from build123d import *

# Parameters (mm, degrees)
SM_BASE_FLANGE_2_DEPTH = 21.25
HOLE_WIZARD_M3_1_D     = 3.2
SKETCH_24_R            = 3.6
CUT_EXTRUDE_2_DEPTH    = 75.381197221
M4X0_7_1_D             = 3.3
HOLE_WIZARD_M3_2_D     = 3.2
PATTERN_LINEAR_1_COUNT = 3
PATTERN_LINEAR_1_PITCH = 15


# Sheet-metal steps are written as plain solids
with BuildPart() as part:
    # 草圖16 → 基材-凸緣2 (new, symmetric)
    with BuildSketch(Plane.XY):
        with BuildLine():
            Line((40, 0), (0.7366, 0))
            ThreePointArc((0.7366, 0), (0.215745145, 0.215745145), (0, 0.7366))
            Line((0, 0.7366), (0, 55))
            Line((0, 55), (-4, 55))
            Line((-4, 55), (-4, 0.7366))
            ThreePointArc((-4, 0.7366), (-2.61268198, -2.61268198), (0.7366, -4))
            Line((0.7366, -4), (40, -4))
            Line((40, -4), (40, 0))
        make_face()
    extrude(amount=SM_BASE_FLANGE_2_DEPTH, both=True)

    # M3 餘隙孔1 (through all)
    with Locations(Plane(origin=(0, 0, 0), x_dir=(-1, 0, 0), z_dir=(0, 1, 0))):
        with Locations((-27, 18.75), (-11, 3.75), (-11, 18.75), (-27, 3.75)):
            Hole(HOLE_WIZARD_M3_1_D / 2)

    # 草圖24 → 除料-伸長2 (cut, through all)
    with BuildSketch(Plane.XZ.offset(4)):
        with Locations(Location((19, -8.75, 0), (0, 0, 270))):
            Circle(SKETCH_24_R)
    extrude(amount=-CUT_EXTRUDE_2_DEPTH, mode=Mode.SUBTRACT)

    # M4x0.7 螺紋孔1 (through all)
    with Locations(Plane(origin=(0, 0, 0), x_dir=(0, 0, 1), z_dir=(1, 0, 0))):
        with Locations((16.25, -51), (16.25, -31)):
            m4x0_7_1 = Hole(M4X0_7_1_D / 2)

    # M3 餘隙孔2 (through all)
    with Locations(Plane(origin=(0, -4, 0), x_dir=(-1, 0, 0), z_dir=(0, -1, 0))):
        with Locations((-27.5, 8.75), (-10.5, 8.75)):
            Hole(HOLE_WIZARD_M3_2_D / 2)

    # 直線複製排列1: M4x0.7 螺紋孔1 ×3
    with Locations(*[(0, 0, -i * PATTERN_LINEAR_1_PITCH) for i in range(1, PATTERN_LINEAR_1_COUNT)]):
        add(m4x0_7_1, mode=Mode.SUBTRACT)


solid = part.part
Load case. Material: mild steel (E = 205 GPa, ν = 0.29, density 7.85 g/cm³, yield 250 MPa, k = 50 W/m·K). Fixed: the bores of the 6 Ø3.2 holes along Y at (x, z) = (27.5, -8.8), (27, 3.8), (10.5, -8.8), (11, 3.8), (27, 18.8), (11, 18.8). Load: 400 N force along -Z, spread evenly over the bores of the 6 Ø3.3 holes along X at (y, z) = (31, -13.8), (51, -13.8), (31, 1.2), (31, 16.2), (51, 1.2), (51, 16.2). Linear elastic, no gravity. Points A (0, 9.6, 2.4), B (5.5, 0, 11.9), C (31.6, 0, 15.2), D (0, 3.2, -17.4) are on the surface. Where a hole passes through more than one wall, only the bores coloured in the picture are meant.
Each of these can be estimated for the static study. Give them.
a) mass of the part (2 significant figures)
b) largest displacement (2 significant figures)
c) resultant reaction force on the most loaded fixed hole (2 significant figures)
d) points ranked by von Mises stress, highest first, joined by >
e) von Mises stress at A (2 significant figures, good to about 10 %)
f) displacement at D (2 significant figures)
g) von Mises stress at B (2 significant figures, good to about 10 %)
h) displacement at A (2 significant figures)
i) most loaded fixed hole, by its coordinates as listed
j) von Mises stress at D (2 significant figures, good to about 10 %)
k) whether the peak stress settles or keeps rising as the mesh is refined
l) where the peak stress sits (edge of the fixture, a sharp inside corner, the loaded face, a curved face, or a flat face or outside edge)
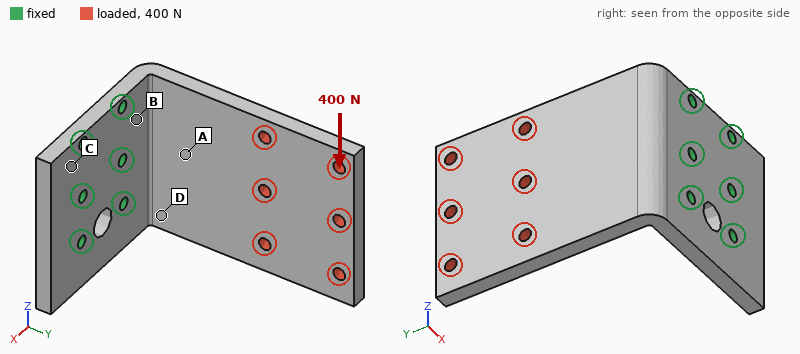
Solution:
130 g
65 µm
720 N
B > D > A > C
20 MPa
18 µm
53 MPa
12 µm
(10.5, -8.8)
39 MPa
keeps rising
edge of the fixture
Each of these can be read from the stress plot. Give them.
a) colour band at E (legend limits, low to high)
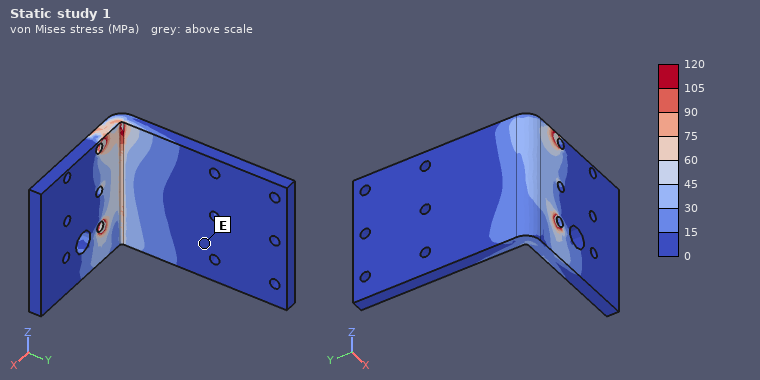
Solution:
0 to 15 MPa
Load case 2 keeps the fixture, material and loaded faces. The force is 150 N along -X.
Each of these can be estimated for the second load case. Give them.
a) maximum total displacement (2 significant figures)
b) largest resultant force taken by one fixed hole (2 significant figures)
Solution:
0.22 mm
89 N
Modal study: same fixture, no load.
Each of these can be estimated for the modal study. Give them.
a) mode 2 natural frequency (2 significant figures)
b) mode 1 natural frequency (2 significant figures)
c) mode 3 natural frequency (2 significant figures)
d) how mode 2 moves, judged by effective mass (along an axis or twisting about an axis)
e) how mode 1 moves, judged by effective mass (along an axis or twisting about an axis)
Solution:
2100 Hz
780 Hz
3100 Hz
along Z
along X
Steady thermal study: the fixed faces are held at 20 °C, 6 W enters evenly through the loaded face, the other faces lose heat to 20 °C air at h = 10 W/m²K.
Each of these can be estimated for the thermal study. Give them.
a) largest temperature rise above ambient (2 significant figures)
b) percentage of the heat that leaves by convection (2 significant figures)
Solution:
34 K
21 %
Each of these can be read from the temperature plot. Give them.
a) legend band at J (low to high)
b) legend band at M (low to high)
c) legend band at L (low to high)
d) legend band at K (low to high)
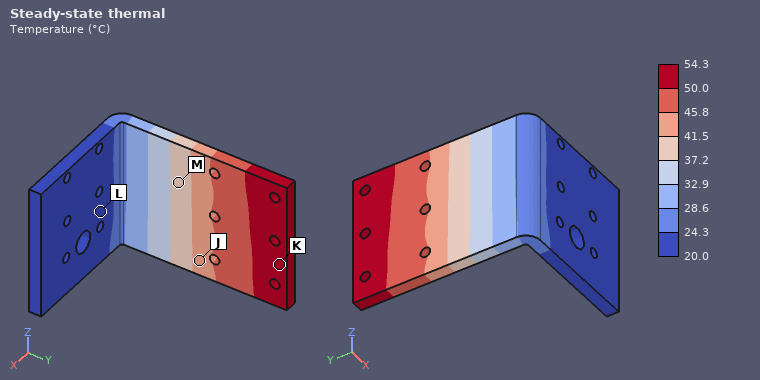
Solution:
41.5 to 45.8 °C
37.2 to 41.5 °C
20.0 to 24.3 °C
50.0 to 54.3 °C
